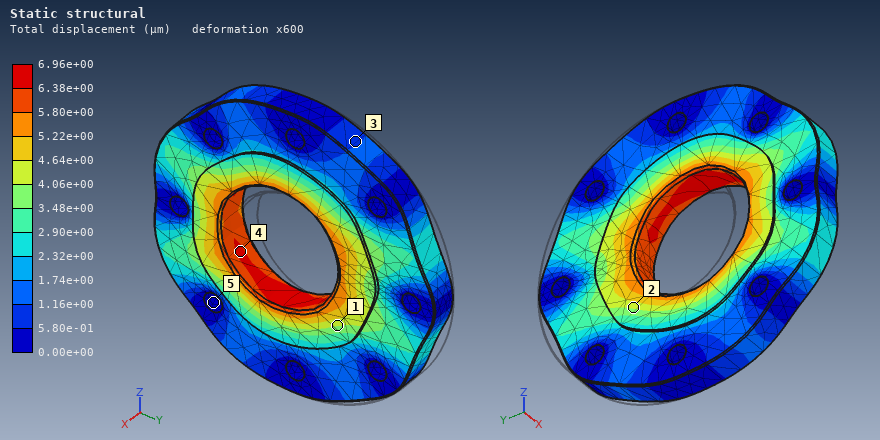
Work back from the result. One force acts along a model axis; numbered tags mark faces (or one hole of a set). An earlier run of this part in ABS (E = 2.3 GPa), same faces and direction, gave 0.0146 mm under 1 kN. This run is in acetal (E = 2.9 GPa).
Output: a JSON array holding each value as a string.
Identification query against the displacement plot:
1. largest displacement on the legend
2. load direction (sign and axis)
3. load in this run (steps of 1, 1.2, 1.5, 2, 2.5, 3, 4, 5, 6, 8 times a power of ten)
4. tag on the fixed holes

["6.96e+00 µm", "-Y", "600 N", "5"]
